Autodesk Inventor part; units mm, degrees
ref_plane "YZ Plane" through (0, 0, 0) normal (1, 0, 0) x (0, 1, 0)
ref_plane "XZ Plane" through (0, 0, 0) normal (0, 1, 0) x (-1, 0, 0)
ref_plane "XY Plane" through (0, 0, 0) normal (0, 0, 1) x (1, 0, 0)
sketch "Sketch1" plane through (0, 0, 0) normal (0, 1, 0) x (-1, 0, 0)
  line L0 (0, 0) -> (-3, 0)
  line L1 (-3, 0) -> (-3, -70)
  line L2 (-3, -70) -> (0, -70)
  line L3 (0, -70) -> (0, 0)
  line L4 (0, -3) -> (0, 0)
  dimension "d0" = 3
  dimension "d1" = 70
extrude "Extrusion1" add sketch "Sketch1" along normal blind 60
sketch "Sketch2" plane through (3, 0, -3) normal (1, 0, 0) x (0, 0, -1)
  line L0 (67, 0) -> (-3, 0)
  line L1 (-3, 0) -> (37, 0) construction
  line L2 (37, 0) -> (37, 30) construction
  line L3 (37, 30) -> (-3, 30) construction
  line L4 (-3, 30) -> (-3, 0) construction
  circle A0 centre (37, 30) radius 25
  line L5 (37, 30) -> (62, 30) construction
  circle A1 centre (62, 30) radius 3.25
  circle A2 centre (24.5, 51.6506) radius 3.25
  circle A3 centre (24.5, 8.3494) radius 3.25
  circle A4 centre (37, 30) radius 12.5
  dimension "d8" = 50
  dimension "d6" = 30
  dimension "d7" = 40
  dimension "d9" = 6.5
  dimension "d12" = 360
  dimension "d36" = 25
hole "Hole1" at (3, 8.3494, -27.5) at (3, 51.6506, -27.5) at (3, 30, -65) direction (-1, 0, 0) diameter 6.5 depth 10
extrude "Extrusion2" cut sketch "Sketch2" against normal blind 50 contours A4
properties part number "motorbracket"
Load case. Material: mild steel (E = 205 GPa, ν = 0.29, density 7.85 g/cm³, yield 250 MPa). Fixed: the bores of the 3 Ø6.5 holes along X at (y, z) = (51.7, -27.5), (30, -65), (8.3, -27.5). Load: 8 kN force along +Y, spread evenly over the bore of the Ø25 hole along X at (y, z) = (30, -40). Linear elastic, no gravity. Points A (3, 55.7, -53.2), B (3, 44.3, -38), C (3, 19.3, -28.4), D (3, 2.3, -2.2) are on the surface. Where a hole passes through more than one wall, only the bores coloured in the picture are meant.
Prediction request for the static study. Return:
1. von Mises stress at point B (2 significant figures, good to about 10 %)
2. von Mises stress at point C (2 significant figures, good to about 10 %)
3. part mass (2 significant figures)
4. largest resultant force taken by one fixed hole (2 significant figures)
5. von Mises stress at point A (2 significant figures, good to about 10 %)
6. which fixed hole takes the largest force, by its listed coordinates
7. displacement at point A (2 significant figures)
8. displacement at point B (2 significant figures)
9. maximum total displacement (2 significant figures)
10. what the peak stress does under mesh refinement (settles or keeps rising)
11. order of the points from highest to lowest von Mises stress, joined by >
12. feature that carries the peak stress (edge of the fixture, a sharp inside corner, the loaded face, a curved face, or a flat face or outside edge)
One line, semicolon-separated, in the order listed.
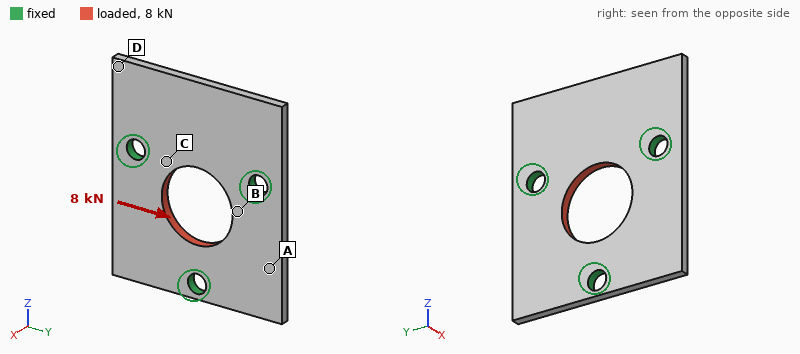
39 MPa; 55 MPa; 85 g; 3.0 kN; 24 MPa; (30, -65); 4.7 µm; 4.6 µm; 6.5 µm; keeps rising; C > B > A > D; edge of the fixture
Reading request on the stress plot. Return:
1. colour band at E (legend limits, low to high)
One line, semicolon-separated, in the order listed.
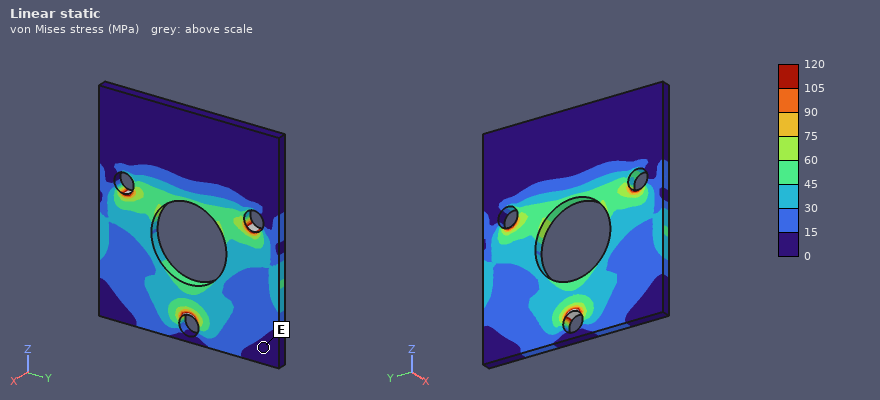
0 to 15 MPa
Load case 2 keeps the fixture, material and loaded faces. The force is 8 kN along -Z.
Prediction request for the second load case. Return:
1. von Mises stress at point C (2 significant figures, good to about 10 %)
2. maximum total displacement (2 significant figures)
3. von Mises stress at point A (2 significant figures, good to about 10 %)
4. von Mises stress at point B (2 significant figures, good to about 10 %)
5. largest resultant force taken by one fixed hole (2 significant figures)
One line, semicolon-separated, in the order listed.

32 MPa; 6.0 µm; 14 MPa; 48 MPa; 2.9 kN
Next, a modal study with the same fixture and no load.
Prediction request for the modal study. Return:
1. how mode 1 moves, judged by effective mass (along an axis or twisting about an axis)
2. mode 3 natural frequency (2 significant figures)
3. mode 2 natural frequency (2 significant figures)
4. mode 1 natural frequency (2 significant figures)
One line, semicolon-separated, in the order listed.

along X; 4300 Hz; 4300 Hz; 3200 Hz
